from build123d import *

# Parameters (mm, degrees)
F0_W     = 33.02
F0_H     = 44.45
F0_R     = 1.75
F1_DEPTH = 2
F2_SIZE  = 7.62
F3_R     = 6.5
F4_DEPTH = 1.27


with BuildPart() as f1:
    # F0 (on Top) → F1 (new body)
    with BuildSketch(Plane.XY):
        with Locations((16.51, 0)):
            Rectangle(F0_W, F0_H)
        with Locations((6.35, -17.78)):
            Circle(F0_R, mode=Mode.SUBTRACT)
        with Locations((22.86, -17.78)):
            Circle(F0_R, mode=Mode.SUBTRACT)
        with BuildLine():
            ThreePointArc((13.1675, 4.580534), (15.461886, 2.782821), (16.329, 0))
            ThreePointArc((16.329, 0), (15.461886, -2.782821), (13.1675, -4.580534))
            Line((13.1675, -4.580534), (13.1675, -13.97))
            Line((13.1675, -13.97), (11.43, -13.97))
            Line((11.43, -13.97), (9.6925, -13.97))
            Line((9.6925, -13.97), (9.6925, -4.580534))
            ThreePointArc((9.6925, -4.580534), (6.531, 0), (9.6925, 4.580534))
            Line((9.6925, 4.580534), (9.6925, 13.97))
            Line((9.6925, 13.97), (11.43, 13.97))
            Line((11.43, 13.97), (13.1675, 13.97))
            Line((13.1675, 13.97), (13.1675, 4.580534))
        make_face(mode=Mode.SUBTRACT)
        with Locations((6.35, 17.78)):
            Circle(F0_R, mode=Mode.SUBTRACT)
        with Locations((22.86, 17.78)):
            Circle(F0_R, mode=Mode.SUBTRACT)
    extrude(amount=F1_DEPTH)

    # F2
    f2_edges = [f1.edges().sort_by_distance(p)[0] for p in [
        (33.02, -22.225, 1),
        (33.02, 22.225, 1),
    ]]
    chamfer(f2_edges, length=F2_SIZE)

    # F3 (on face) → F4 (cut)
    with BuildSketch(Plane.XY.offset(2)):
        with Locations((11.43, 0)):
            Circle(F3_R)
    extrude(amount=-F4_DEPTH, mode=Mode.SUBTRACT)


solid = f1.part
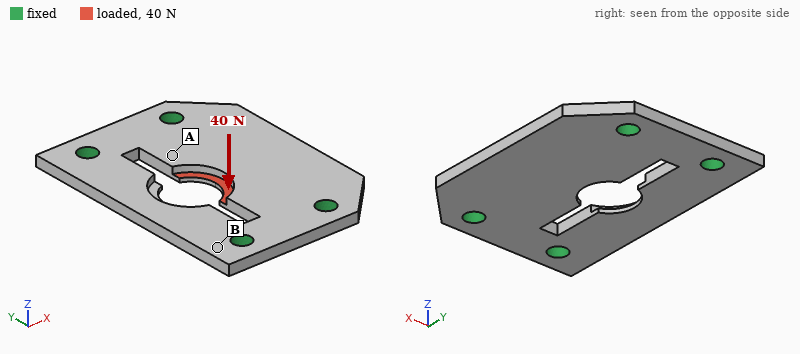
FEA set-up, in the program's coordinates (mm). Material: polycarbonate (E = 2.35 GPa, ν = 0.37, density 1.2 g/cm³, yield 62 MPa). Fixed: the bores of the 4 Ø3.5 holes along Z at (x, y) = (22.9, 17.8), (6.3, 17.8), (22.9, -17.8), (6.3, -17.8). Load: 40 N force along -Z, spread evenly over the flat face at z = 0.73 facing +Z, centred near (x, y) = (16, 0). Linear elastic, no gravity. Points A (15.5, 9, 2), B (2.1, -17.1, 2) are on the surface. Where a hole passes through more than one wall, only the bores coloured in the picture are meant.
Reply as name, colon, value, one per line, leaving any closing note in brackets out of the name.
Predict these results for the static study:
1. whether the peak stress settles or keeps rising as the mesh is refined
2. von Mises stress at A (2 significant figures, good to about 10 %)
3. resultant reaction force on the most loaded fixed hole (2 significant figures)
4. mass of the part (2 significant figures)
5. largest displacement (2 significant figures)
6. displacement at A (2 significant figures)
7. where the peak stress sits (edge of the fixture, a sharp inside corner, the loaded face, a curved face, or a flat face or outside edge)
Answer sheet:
whether the peak stress settles or keeps rising as the mesh is refined: keeps rising
von Mises stress at A: 11 MPa
resultant reaction force on the most loaded fixed hole: 15 N
mass of the part: 2.9 g
largest displacement: 0.62 mm
displacement at A: 0.29 mm
where the peak stress sits: edge of the fixture
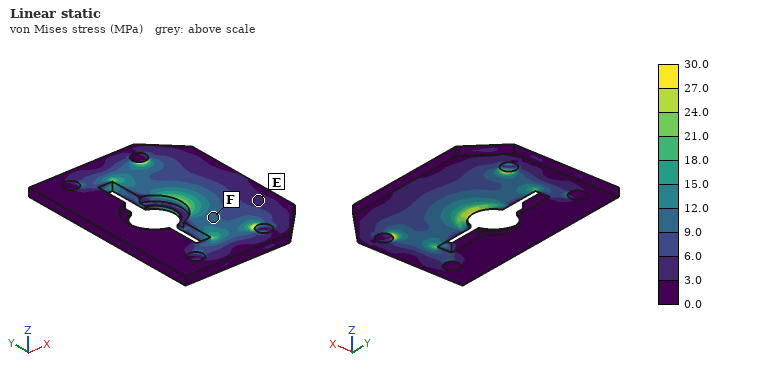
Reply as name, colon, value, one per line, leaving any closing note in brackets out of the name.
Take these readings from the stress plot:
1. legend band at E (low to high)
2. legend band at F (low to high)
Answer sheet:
legend band at E: 3.0 to 6.0 MPa
legend band at F: 9.0 to 12.0 MPa
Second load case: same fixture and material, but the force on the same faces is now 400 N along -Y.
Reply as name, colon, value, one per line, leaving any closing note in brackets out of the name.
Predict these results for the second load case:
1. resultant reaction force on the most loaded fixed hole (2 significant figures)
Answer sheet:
resultant reaction force on the most loaded fixed hole: 180 N
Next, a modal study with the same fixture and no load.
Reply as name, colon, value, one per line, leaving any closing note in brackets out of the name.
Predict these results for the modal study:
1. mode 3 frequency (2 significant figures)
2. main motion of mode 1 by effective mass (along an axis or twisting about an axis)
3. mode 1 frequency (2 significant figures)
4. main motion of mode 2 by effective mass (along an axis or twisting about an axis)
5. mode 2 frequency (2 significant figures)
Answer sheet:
mode 3 frequency: 3200 Hz
main motion of mode 1 by effective mass: along Z
mode 1 frequency: 2200 Hz
main motion of mode 2 by effective mass: along Z
mode 2 frequency: 2600 Hz
